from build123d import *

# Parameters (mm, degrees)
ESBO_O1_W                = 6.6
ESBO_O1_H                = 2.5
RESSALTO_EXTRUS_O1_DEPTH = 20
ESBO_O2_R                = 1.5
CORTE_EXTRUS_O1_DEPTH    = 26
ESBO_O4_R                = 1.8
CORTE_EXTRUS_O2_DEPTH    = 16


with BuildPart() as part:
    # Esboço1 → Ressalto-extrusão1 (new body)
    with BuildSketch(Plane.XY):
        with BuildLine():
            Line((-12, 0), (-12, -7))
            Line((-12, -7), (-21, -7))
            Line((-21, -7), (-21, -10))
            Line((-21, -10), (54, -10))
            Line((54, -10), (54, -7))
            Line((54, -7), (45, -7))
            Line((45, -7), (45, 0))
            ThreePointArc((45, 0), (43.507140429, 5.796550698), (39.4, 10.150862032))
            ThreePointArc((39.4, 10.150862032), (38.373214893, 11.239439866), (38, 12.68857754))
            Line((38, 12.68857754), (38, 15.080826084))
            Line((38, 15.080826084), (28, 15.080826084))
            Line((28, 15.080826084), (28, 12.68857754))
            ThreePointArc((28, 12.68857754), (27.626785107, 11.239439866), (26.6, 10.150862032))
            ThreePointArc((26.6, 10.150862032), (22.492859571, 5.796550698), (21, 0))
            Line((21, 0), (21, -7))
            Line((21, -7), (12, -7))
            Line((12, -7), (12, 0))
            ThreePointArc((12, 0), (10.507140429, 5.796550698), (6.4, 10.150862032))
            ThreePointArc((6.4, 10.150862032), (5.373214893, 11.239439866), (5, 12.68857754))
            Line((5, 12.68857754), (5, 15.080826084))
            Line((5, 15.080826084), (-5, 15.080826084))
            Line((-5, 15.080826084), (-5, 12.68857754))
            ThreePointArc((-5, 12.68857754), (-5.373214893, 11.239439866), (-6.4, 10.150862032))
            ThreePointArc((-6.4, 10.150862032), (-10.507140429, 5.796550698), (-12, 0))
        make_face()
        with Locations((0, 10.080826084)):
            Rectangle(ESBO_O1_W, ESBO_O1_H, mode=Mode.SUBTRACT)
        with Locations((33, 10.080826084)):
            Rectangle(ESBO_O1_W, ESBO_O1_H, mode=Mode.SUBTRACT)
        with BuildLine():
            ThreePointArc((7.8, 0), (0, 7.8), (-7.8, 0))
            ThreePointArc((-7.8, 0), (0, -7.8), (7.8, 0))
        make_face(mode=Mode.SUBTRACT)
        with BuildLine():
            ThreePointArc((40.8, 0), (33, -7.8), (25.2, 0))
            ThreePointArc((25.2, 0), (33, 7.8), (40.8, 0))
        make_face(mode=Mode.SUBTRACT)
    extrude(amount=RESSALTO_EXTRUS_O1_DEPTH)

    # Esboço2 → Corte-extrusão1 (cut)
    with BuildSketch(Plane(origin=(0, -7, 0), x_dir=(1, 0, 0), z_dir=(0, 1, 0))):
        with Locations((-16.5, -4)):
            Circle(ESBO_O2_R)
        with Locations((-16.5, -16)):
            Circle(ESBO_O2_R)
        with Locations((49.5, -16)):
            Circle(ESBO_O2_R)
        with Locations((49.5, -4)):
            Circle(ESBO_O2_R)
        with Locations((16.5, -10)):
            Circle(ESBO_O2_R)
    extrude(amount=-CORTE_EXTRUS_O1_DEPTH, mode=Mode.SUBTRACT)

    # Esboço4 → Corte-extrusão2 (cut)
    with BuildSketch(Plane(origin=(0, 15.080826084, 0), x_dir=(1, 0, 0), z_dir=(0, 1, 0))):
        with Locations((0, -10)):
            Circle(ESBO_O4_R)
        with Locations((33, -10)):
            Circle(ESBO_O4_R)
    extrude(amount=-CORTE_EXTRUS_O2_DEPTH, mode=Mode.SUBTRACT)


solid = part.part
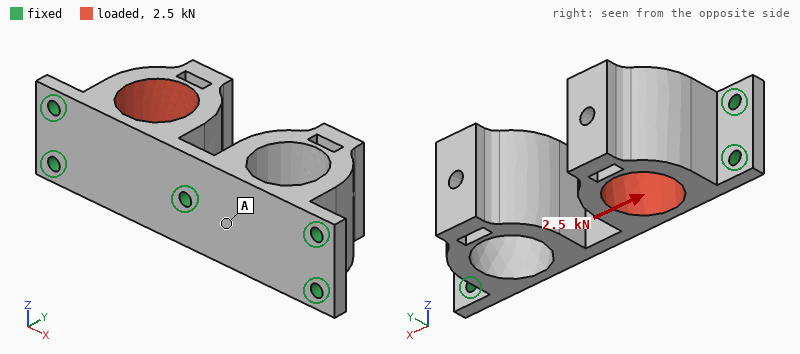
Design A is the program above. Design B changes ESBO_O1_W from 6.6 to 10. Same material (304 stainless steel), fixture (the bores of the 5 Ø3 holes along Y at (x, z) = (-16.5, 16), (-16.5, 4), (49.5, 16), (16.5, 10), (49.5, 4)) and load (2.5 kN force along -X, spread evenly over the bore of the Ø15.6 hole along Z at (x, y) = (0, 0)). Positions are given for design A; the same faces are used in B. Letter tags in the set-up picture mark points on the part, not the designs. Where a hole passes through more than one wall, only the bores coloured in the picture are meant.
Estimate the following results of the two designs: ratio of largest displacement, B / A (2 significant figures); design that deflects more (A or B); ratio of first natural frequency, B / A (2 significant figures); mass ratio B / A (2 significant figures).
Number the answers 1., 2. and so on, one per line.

1. 1.3
2. B
3. 1.0
4. 0.97
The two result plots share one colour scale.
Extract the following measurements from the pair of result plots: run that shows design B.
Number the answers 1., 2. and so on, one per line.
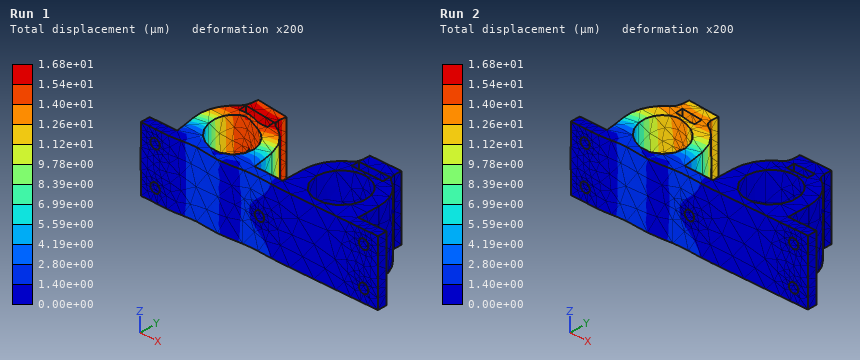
1. Run 1
